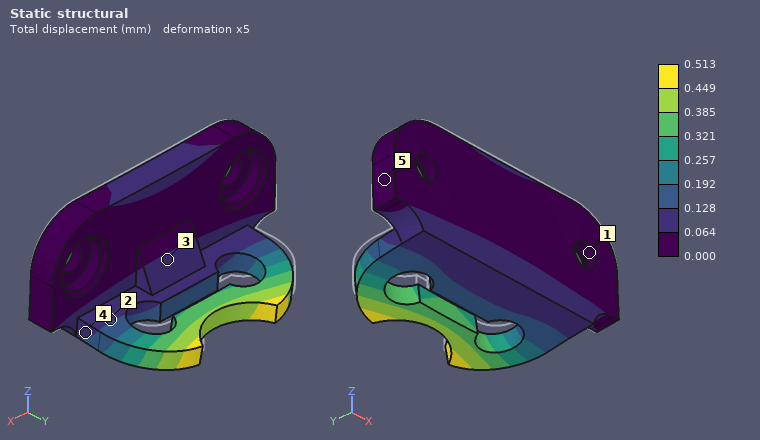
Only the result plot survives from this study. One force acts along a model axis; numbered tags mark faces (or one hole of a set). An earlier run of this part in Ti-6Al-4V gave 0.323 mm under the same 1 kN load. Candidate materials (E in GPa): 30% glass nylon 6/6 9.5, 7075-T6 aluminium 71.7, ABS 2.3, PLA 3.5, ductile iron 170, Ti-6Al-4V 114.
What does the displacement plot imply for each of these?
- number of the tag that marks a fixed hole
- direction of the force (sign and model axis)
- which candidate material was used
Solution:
1
-Z
7075-T6 aluminium
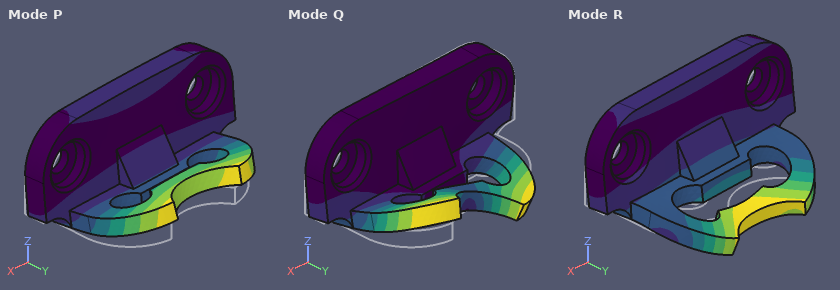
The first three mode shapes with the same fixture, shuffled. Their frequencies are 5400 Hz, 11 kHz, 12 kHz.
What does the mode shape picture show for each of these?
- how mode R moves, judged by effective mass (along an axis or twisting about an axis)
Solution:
along Y
